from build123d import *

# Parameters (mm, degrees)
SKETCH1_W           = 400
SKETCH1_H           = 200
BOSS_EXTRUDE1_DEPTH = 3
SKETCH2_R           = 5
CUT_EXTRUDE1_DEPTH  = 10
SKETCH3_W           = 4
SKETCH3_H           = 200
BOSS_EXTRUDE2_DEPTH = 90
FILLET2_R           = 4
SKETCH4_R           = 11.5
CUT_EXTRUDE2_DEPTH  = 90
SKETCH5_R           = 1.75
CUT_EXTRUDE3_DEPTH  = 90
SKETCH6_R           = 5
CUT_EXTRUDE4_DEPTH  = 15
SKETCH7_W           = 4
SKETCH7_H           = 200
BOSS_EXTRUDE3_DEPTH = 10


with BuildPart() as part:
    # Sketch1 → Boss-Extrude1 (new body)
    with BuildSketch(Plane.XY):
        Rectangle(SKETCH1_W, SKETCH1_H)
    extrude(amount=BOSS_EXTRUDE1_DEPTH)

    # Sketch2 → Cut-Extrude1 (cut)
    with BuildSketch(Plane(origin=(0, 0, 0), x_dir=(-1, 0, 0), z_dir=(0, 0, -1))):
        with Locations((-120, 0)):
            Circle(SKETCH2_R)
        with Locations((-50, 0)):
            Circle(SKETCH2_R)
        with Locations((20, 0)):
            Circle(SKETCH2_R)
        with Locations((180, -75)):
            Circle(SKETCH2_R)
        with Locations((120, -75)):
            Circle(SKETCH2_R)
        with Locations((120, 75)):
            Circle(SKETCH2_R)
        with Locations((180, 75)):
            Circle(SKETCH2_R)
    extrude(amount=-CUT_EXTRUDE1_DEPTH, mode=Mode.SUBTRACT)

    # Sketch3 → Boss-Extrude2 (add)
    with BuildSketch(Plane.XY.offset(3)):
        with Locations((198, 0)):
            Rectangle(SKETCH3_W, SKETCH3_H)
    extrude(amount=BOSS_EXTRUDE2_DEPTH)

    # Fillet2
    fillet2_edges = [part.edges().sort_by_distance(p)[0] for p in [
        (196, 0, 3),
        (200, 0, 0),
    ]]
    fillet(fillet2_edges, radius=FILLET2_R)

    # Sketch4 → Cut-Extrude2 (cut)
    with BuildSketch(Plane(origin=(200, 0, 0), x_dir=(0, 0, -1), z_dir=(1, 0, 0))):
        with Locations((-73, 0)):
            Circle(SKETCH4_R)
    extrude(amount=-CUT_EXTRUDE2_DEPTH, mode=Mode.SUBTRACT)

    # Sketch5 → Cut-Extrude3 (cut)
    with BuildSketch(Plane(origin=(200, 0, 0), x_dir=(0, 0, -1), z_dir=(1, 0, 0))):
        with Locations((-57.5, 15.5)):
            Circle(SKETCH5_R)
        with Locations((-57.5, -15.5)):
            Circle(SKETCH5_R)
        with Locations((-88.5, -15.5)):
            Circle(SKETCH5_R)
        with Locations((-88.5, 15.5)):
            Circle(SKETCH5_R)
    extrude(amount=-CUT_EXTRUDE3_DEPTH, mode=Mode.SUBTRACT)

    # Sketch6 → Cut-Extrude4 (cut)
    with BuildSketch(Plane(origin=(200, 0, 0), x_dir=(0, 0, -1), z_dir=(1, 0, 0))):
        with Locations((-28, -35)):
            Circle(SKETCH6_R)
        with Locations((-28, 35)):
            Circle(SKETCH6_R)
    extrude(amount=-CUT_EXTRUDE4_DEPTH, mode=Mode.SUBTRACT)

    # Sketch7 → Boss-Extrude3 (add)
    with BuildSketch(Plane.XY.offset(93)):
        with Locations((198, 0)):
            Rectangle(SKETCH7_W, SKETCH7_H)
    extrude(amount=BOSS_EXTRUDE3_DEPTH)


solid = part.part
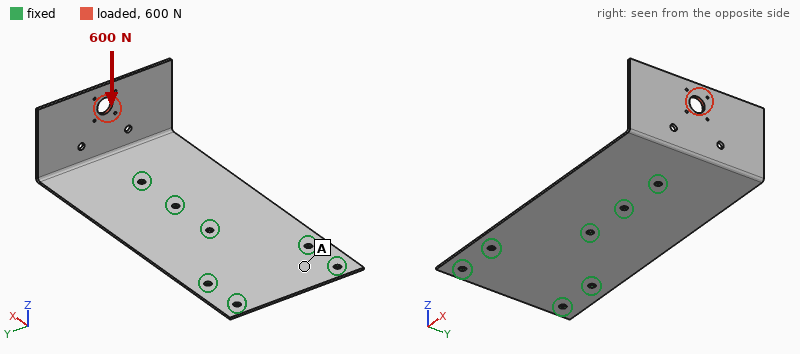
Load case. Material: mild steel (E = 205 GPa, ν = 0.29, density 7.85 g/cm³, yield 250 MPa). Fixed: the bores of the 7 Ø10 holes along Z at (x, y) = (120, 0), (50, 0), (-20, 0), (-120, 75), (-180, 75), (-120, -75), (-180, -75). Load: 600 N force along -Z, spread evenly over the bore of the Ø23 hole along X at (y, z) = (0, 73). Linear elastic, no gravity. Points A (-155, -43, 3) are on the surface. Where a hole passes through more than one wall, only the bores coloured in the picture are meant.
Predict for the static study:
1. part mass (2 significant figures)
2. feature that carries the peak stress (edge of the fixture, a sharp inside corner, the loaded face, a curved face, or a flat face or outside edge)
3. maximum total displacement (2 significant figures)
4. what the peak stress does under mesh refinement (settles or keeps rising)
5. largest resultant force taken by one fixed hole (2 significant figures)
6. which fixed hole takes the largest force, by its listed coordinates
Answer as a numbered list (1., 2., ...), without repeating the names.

1. 2.5 kg
2. edge of the fixture
3. 2.9 mm
4. keeps rising
5. 890 N
6. (120, 0)
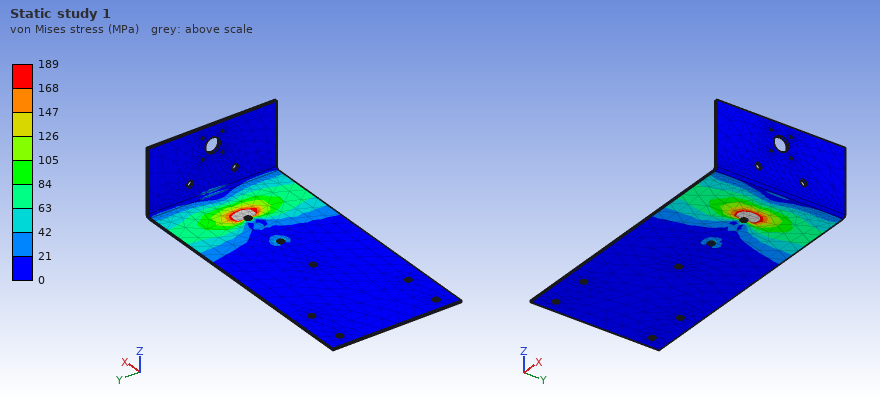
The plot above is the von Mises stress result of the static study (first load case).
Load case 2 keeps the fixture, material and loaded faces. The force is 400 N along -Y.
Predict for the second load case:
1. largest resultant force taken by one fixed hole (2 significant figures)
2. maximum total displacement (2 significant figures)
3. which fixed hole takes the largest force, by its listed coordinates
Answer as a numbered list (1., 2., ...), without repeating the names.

1. 520 N
2. 2.0 mm
3. (120, 0)
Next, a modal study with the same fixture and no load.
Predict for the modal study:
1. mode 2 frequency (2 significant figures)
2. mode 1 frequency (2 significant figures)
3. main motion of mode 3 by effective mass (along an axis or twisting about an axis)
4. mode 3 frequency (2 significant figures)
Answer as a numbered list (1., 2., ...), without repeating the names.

1. 100 Hz
2. 85 Hz
3. along Z
4. 240 Hz
